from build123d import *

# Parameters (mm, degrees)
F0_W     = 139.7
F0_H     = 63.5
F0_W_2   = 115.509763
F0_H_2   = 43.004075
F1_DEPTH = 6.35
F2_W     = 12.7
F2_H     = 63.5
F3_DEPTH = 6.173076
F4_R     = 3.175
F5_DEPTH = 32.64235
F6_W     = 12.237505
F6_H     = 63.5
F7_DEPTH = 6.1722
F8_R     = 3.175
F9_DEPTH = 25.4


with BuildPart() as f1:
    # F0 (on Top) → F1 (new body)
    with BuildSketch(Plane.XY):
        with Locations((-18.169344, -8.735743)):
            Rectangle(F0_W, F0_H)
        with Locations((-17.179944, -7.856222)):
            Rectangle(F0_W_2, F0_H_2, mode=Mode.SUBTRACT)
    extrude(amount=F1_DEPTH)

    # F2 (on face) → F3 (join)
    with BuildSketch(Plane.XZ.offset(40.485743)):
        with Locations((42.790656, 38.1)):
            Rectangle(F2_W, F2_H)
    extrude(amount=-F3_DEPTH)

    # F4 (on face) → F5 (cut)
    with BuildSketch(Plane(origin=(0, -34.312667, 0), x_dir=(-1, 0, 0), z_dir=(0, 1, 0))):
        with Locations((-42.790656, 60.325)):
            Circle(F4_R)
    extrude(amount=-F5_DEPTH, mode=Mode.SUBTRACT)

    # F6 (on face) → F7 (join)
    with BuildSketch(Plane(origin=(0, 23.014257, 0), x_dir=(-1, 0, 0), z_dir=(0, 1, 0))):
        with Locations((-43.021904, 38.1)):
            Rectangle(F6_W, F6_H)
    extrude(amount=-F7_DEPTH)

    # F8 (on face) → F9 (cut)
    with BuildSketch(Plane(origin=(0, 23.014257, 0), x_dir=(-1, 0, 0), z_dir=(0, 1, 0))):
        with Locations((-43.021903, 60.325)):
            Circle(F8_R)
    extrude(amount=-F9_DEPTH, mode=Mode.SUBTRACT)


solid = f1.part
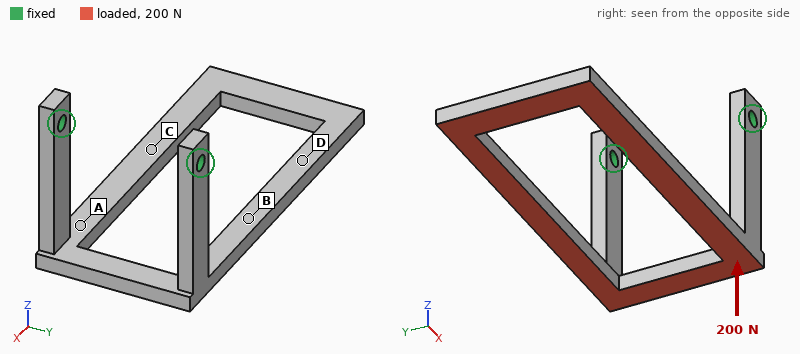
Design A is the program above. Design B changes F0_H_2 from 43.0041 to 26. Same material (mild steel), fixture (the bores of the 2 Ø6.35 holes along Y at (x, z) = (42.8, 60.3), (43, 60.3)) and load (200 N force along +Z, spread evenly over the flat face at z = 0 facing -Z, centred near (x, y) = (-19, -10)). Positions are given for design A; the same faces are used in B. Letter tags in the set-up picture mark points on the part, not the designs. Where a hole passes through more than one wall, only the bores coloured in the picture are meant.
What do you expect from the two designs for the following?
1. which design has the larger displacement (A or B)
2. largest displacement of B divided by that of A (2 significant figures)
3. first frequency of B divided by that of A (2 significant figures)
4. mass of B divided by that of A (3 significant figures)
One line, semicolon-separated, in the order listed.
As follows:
A; 0.67; 1.0; 1.36
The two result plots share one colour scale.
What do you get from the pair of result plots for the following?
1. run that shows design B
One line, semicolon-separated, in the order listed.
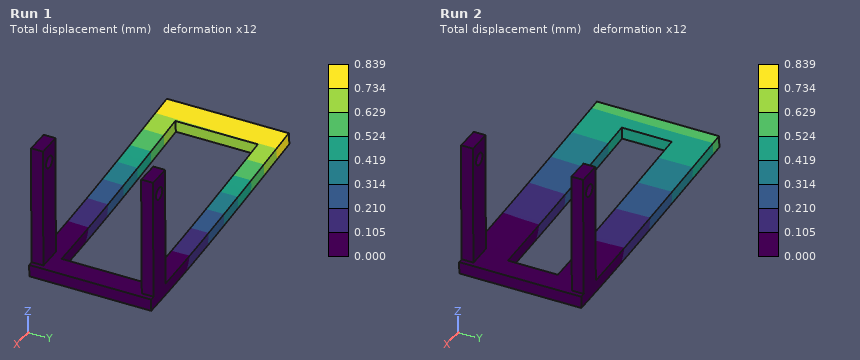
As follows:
Run 2
